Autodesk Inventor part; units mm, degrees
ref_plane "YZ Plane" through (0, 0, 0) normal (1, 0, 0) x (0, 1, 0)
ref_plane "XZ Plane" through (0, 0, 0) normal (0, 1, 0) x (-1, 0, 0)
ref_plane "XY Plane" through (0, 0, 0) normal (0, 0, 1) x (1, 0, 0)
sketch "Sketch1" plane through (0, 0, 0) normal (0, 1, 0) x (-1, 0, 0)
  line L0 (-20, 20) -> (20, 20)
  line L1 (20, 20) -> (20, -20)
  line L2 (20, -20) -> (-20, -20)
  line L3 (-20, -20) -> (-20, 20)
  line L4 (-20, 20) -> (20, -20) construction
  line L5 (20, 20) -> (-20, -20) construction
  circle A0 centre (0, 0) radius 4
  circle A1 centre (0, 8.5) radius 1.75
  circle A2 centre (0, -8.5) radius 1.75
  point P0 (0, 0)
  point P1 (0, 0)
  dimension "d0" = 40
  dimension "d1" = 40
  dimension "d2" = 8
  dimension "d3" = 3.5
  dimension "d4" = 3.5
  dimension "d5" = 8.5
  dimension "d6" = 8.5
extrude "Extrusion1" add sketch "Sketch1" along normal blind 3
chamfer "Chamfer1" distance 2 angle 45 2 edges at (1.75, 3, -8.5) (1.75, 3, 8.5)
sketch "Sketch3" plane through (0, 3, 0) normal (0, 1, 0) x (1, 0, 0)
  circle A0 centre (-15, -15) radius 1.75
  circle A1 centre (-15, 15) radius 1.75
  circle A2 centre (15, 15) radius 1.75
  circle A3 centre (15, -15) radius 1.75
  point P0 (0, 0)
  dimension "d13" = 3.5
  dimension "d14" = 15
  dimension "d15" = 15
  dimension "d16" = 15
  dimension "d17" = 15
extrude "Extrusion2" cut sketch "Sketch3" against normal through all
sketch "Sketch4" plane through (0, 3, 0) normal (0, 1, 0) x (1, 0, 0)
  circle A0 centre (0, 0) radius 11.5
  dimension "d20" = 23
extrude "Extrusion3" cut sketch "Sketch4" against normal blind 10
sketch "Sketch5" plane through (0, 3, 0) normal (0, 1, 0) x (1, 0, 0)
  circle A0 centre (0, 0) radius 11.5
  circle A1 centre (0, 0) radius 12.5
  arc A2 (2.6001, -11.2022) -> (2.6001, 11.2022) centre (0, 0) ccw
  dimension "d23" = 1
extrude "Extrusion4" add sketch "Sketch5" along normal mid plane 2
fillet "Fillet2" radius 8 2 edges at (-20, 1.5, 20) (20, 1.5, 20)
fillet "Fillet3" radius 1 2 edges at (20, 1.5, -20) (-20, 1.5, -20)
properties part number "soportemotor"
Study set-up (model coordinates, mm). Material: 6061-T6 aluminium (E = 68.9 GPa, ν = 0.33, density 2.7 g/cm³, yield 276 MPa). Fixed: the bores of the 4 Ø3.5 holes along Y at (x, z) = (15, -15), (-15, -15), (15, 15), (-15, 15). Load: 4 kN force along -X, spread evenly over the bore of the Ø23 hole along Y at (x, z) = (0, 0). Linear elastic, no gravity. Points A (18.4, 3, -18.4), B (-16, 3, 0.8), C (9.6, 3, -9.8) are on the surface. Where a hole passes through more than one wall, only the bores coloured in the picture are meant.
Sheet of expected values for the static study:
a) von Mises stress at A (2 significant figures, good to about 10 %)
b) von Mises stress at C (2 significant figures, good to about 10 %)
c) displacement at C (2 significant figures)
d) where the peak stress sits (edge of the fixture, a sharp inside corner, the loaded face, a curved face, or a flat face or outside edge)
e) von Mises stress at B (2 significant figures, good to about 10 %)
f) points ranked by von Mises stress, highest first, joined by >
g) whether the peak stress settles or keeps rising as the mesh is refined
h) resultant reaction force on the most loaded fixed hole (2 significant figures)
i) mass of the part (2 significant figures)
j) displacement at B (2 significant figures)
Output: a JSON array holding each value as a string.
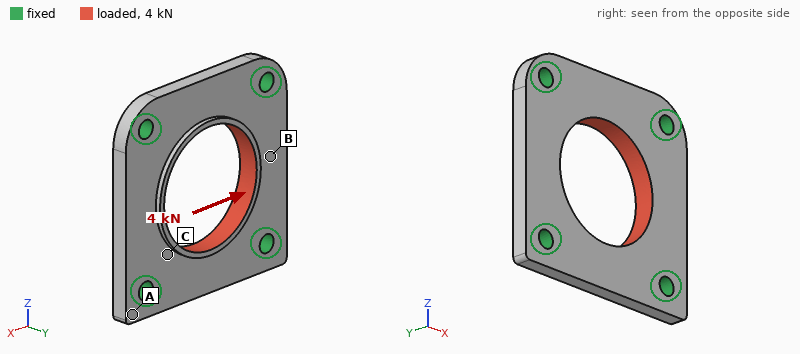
["9.8 MPa", "35 MPa", "5.9 µm", "edge of the fixture", "19 MPa", "C > B > A", "keeps rising", "1.0 kN", "9.3 g", "13 µm"]
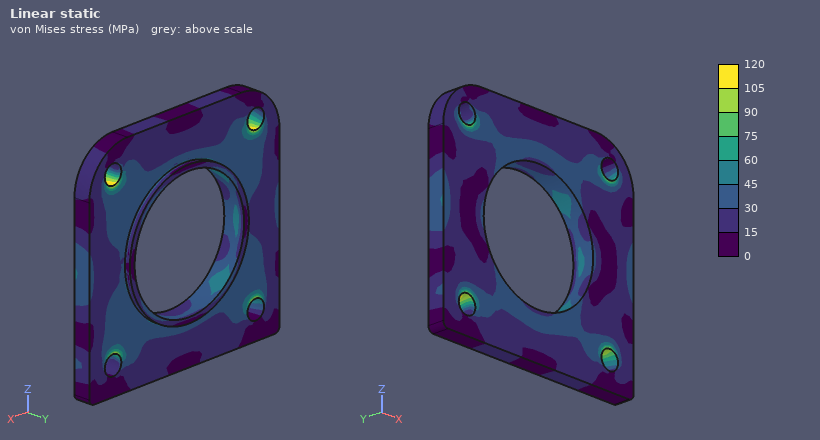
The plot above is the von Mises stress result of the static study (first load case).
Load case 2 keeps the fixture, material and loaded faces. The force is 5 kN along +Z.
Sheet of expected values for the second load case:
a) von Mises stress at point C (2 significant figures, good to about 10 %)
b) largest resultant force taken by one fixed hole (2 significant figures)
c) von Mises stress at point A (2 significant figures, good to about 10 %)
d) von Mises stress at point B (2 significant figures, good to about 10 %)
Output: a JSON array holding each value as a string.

["43 MPa", "1.3 kN", "12 MPa", "28 MPa"]
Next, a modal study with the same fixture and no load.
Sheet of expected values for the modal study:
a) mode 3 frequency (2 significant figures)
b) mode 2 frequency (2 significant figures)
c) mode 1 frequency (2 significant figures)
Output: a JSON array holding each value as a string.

["19 kHz", "19 kHz", "19 kHz"]
